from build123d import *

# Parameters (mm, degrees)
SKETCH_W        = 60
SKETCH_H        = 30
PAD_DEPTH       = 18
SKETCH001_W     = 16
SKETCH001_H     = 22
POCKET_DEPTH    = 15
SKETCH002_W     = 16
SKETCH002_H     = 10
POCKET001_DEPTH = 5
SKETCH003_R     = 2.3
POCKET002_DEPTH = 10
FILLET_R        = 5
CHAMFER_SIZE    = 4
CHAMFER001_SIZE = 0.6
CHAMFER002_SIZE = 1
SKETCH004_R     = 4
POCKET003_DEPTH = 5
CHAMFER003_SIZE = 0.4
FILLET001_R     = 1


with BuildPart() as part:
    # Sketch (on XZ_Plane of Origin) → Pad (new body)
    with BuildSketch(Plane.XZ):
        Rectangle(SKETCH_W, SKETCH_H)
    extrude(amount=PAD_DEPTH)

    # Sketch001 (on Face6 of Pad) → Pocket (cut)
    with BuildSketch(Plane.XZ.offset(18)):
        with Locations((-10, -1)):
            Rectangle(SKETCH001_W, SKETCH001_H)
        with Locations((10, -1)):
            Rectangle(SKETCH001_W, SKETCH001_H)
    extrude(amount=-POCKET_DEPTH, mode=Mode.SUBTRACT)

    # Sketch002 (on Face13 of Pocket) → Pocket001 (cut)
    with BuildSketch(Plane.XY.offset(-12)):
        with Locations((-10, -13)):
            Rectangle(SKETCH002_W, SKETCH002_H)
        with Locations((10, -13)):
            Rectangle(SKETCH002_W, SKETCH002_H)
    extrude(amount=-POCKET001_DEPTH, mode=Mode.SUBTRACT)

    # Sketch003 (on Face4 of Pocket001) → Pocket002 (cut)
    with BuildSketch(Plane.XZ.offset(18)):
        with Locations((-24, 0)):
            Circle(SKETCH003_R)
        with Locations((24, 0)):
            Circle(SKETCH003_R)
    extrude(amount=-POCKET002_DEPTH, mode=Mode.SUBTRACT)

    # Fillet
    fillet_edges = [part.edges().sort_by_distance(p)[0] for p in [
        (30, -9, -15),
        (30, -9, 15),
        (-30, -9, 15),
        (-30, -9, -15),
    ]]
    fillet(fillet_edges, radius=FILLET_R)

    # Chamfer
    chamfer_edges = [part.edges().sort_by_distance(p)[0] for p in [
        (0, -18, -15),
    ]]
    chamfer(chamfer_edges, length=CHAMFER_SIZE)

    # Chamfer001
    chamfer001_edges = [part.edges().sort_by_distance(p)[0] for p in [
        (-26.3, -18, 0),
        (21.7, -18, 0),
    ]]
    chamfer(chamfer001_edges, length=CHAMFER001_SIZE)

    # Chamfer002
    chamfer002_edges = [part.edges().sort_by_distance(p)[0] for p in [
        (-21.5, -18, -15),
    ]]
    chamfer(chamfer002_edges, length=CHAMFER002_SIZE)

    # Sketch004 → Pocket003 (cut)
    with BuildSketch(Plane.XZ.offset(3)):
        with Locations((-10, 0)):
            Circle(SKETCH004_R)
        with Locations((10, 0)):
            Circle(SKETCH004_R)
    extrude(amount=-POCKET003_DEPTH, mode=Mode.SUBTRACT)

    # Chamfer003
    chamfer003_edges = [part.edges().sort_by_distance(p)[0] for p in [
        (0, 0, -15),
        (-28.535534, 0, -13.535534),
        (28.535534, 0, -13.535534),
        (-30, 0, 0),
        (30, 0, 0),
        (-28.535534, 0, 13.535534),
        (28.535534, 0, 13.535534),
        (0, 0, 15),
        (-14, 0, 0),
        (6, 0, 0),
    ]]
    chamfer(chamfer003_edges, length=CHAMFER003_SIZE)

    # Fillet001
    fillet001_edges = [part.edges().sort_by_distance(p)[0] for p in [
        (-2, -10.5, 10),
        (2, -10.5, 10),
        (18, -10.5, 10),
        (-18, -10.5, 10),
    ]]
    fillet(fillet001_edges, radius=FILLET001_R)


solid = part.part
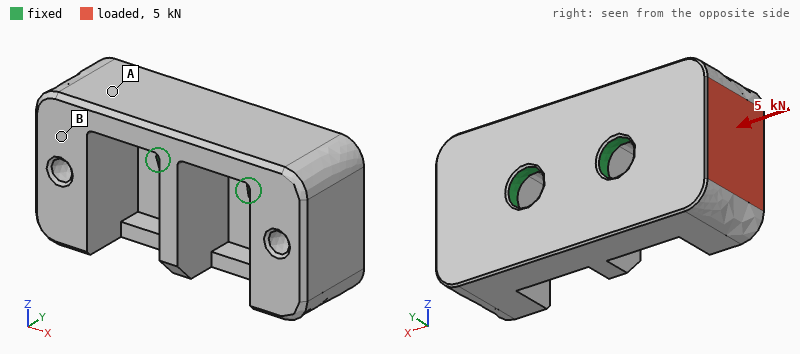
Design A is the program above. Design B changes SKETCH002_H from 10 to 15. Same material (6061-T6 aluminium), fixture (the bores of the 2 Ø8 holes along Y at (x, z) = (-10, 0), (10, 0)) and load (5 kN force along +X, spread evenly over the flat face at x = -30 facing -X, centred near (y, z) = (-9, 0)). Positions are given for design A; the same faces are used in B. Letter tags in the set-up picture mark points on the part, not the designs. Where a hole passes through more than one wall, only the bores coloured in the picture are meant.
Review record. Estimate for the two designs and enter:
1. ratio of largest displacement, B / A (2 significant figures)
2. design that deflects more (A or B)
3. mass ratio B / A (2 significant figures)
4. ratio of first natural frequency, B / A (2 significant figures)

1.2
B
0.99
1.00
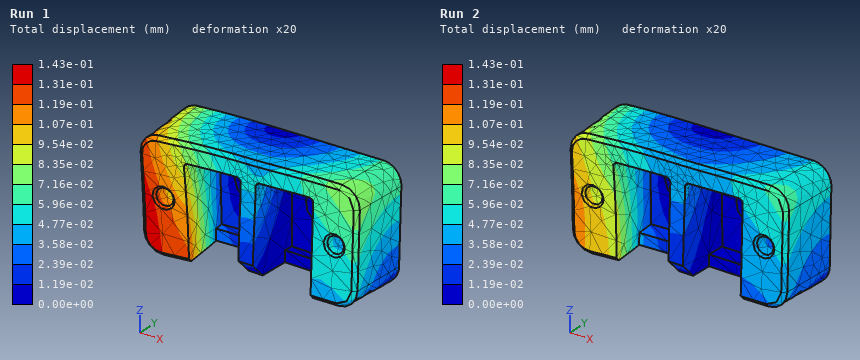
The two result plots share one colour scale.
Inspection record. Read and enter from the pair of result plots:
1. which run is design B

Run 1
